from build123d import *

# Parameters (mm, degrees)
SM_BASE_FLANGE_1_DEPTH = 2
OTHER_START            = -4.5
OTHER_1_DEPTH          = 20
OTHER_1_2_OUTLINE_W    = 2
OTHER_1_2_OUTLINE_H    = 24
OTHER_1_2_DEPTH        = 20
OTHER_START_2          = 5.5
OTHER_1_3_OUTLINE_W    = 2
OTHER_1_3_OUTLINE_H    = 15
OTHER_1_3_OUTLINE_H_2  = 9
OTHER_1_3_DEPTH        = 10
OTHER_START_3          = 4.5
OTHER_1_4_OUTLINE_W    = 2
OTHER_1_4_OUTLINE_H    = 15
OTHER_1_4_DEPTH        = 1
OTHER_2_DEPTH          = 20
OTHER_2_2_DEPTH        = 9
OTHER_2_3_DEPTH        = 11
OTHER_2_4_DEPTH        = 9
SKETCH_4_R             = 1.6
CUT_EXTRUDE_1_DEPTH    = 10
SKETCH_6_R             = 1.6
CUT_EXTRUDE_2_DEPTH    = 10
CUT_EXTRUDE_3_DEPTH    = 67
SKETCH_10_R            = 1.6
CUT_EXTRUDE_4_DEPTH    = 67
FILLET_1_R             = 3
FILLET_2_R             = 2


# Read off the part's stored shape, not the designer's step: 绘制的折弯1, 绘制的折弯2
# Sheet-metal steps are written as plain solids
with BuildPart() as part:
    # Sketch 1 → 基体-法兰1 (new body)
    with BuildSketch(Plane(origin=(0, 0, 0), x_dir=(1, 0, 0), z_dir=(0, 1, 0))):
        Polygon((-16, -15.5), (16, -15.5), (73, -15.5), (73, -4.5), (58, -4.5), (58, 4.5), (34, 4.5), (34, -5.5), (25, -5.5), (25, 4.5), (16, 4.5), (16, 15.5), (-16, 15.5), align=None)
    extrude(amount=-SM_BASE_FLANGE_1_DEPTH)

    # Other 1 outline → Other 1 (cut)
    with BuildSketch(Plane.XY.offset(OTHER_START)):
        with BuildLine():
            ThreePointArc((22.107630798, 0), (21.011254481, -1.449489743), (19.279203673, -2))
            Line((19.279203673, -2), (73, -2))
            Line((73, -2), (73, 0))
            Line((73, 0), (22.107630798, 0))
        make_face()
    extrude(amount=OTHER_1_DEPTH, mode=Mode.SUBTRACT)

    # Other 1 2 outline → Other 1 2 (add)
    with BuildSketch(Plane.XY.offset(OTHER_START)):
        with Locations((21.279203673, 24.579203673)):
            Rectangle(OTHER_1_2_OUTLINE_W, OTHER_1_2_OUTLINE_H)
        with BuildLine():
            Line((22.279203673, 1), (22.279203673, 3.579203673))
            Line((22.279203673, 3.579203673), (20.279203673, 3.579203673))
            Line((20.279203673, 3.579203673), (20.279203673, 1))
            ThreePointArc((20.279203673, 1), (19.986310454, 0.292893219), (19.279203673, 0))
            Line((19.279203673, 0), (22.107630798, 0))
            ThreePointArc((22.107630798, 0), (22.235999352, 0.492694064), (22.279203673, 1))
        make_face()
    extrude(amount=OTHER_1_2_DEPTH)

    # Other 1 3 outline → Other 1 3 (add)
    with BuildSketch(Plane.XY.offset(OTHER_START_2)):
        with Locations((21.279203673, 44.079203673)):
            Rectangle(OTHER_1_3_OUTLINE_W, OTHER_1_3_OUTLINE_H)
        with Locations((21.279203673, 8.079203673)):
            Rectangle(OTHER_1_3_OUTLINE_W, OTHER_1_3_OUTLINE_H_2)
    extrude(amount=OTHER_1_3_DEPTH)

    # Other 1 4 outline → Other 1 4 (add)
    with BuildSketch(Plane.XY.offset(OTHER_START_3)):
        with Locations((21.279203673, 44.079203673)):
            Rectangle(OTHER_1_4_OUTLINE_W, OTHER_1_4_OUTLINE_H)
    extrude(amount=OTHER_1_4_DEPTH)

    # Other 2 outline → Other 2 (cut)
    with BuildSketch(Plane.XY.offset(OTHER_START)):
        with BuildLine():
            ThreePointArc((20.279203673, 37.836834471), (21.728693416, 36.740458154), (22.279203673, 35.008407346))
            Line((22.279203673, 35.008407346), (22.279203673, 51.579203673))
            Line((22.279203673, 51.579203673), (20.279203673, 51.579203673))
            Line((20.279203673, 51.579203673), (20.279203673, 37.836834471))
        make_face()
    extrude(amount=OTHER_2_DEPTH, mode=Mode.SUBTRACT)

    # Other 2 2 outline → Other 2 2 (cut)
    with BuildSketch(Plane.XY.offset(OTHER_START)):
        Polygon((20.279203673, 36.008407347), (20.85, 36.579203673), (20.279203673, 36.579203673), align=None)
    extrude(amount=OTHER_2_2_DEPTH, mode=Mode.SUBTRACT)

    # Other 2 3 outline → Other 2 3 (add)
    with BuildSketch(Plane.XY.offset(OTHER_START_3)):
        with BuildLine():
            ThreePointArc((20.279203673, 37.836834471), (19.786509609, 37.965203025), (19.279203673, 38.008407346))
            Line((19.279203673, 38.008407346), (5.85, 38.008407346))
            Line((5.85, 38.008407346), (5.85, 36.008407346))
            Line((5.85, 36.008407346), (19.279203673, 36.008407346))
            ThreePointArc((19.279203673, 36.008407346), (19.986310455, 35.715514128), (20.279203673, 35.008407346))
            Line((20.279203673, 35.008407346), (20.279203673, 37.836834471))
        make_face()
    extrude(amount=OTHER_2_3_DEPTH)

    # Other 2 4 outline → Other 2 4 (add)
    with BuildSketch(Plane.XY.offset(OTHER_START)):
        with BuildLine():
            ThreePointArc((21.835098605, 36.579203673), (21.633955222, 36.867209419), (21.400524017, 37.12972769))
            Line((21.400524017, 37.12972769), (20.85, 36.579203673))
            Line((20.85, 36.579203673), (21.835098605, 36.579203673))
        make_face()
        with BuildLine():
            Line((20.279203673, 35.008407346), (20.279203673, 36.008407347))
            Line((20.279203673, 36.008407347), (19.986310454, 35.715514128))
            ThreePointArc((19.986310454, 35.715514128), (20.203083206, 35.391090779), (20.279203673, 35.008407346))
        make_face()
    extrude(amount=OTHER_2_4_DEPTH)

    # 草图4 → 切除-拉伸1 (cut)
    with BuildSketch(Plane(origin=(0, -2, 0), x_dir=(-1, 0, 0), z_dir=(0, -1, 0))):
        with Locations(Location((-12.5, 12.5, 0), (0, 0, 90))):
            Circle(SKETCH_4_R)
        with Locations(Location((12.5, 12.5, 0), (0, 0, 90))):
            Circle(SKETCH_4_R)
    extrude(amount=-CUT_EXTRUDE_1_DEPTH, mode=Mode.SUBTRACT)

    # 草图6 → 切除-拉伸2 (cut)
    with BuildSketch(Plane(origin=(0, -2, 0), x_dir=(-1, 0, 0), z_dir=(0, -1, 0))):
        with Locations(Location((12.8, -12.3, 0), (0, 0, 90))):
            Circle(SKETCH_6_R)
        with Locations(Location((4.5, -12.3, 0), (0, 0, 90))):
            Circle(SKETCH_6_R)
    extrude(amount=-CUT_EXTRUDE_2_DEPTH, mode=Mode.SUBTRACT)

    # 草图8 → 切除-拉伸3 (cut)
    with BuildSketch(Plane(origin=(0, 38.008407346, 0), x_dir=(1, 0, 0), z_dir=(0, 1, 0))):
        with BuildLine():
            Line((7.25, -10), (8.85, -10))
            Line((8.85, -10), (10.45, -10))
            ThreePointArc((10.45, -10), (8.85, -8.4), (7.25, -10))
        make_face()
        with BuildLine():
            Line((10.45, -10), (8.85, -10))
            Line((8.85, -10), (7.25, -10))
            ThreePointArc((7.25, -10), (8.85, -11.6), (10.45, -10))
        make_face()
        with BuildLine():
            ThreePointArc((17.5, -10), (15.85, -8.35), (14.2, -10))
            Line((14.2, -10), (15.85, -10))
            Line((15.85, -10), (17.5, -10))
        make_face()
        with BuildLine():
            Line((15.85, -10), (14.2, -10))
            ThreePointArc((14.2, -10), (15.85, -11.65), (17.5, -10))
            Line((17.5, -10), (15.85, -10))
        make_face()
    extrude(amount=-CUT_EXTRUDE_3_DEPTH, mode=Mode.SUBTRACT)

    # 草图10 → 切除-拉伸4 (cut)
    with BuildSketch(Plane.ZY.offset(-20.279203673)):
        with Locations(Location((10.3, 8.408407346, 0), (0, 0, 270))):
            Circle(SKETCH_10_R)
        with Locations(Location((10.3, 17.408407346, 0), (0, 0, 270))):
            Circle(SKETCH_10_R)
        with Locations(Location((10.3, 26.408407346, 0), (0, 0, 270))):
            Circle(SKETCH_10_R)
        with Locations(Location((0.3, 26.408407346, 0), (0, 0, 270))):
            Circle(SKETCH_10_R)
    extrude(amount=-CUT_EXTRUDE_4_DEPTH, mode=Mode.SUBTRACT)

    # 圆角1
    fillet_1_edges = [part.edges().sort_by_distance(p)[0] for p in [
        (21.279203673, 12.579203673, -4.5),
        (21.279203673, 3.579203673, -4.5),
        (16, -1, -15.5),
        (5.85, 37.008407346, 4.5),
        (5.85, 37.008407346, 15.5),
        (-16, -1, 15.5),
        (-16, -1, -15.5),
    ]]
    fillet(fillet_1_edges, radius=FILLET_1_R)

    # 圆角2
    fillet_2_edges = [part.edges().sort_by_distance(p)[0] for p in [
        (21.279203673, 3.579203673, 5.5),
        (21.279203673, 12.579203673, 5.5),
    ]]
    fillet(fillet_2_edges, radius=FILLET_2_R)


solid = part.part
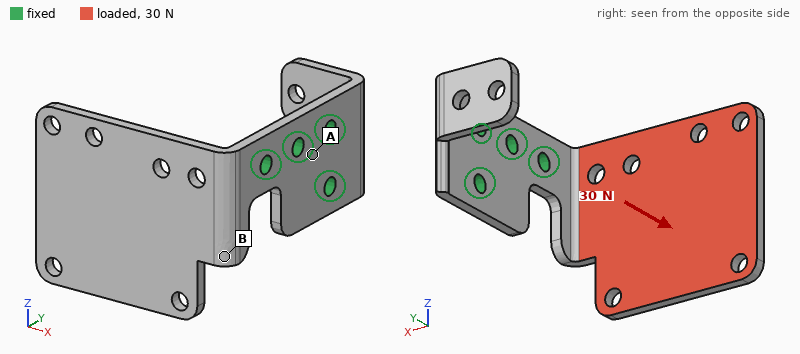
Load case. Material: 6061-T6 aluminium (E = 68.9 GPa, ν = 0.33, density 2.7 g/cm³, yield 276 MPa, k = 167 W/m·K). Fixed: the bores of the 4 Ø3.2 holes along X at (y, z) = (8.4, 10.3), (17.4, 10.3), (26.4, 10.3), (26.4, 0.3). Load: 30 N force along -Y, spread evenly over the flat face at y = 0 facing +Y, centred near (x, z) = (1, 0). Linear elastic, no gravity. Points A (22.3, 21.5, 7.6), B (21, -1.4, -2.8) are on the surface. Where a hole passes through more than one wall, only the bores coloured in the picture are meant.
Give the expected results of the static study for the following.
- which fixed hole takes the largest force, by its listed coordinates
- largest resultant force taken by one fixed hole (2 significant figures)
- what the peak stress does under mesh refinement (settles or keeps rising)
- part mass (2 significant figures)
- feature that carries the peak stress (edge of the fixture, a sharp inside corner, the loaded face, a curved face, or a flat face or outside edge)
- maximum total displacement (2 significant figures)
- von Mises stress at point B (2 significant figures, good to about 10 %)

(8.4, 10.3)
31 N
keeps rising
9.7 g
edge of the fixture
0.67 mm
22 MPa
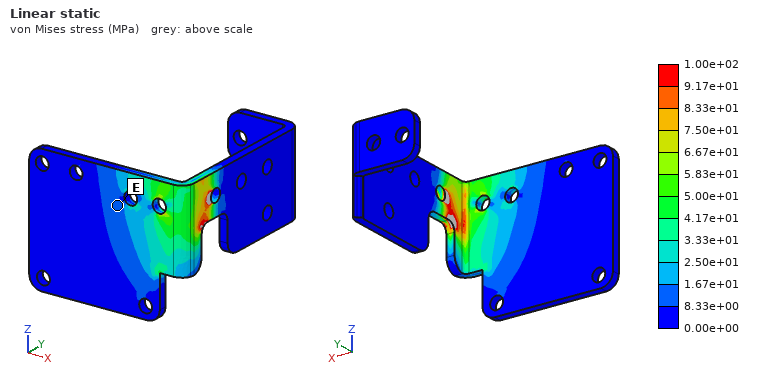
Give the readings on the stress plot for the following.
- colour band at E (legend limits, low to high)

8.33e+00 to 1.67e+01 MPa
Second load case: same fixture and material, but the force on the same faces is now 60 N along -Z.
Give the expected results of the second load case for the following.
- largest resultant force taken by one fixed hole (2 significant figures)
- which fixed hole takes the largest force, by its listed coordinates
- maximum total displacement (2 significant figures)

81 N
(8.4, 10.3)
0.54 mm
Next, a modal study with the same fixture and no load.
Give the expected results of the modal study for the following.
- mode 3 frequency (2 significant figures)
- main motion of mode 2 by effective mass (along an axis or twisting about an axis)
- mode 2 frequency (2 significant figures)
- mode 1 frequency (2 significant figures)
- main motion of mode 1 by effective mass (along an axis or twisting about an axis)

2300 Hz
along Z
870 Hz
570 Hz
along Y
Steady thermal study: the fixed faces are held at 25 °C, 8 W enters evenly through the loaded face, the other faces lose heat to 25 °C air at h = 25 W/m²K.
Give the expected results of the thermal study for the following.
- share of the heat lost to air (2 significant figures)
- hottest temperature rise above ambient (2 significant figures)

15 %
37 K
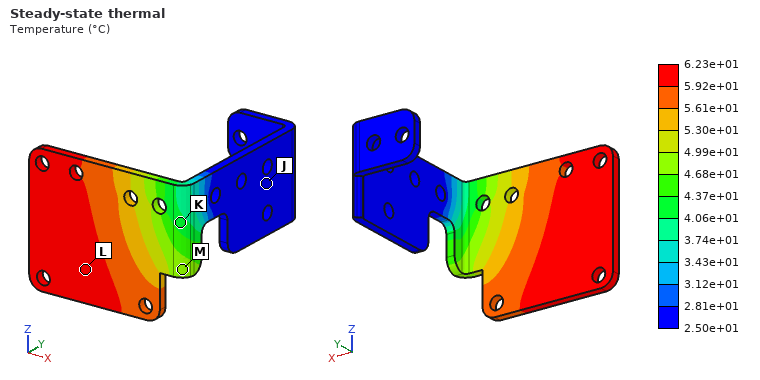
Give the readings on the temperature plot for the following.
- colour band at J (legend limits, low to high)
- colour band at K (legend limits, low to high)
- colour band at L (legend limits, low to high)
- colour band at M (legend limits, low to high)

2.50e+01 to 2.81e+01 °C
4.06e+01 to 4.37e+01 °C
5.92e+01 to 6.23e+01 °C
4.68e+01 to 4.99e+01 °C
